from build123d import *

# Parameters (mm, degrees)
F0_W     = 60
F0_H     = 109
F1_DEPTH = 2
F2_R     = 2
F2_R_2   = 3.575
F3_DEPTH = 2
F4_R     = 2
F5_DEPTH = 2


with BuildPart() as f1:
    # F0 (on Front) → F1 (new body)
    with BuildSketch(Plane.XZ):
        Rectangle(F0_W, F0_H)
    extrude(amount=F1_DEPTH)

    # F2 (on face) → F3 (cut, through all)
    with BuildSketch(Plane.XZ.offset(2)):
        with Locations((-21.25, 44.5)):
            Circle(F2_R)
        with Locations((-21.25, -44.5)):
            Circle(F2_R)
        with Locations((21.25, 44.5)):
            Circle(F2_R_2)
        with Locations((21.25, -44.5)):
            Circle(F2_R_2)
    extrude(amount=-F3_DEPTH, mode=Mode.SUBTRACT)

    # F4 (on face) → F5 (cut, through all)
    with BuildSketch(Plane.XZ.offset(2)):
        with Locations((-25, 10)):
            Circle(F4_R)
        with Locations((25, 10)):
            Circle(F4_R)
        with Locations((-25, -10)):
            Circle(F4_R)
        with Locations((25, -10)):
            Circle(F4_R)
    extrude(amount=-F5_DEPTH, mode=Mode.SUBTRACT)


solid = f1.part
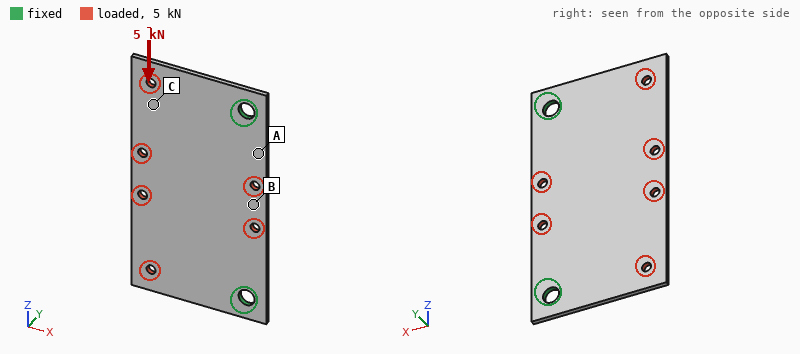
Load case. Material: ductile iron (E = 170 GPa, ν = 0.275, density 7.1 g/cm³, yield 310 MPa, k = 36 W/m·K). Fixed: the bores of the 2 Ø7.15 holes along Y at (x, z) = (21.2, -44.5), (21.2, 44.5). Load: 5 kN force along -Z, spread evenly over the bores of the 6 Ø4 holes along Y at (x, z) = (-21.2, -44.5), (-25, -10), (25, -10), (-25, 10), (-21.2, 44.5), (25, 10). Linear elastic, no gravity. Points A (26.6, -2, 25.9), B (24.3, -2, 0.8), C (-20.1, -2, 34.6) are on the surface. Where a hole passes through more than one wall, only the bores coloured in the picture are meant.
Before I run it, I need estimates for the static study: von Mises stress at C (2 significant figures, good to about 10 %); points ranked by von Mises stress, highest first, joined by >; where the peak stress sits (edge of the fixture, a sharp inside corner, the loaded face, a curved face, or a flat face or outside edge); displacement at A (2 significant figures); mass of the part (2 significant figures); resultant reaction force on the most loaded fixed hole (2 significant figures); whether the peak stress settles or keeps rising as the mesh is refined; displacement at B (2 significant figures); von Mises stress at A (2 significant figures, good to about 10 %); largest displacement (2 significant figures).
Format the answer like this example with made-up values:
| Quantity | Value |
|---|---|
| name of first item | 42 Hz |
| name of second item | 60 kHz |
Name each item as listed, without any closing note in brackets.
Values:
| Quantity | Value |
|---|---|
| von Mises stress at C | 24 MPa |
| points ranked by von Mises stress, highest first, joined by > | A > C > B |
| where the peak stress sits | edge of the fixture |
| displacement at A | 5.0 µm |
| mass of the part | 91 g |
| resultant reaction force on the most loaded fixed hole | 2.9 kN |
| whether the peak stress settles or keeps rising as the mesh is refined | keeps rising |
| displacement at B | 9.2 µm |
| von Mises stress at A | 43 MPa |
| largest displacement | 23 µm |
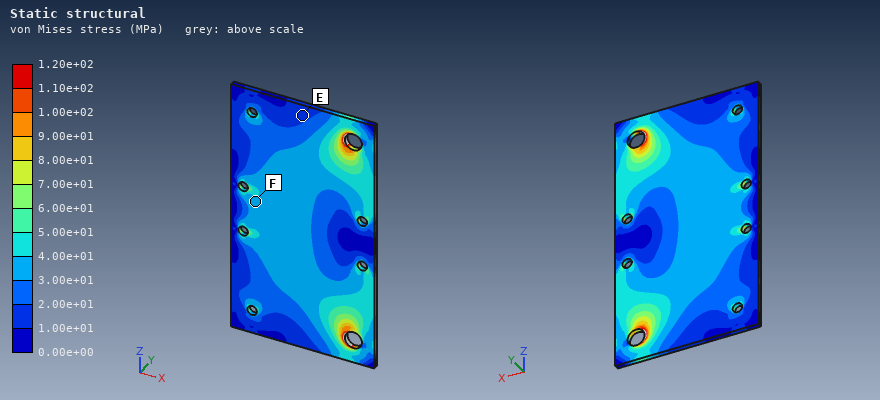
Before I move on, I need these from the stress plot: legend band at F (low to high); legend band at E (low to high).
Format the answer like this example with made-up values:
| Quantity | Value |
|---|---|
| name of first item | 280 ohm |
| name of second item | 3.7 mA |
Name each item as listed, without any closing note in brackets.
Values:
| Quantity | Value |
|---|---|
| legend band at F | 3.00e+01 to 4.00e+01 MPa |
| legend band at E | 1.00e+01 to 2.00e+01 MPa |
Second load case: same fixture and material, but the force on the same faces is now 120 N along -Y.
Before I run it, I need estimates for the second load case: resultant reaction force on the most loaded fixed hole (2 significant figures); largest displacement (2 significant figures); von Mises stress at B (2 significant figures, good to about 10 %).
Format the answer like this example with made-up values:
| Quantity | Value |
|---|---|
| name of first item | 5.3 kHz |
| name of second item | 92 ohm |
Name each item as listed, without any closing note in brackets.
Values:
| Quantity | Value |
|---|---|
| resultant reaction force on the most loaded fixed hole | 60 N |
| largest displacement | 0.36 mm |
| von Mises stress at B | 14 MPa |
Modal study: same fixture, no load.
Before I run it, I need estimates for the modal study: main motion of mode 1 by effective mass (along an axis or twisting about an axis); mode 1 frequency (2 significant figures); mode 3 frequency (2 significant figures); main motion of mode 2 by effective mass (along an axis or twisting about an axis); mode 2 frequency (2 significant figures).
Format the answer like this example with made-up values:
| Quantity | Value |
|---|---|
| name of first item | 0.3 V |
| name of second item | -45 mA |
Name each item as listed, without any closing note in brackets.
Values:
| Quantity | Value |
|---|---|
| main motion of mode 1 by effective mass | along Y |
| mode 1 frequency | 490 Hz |
| mode 3 frequency | 1300 Hz |
| main motion of mode 2 by effective mass | twisting about X |
| mode 2 frequency | 950 Hz |
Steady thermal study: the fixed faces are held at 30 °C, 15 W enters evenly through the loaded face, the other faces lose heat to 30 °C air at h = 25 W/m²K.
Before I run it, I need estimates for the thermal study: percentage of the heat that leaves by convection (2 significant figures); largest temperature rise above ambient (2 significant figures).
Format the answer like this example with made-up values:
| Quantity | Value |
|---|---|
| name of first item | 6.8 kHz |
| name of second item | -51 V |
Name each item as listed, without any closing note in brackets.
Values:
| Quantity | Value |
|---|---|
| percentage of the heat that leaves by convection | 63 % |
| largest temperature rise above ambient | 55 K |
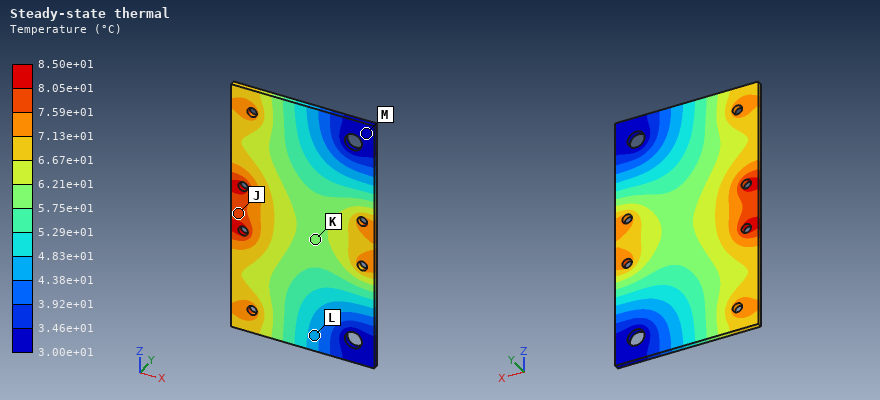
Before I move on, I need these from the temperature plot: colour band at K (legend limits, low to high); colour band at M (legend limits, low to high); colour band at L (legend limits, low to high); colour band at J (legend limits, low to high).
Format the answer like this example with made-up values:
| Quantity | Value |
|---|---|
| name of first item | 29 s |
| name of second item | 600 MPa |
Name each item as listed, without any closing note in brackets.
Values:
| Quantity | Value |
|---|---|
| colour band at K | 5.75e+01 to 6.21e+01 °C |
| colour band at M | 3.00e+01 to 3.46e+01 °C |
| colour band at L | 4.38e+01 to 4.83e+01 °C |
| colour band at J | 7.59e+01 to 8.05e+01 °C |
